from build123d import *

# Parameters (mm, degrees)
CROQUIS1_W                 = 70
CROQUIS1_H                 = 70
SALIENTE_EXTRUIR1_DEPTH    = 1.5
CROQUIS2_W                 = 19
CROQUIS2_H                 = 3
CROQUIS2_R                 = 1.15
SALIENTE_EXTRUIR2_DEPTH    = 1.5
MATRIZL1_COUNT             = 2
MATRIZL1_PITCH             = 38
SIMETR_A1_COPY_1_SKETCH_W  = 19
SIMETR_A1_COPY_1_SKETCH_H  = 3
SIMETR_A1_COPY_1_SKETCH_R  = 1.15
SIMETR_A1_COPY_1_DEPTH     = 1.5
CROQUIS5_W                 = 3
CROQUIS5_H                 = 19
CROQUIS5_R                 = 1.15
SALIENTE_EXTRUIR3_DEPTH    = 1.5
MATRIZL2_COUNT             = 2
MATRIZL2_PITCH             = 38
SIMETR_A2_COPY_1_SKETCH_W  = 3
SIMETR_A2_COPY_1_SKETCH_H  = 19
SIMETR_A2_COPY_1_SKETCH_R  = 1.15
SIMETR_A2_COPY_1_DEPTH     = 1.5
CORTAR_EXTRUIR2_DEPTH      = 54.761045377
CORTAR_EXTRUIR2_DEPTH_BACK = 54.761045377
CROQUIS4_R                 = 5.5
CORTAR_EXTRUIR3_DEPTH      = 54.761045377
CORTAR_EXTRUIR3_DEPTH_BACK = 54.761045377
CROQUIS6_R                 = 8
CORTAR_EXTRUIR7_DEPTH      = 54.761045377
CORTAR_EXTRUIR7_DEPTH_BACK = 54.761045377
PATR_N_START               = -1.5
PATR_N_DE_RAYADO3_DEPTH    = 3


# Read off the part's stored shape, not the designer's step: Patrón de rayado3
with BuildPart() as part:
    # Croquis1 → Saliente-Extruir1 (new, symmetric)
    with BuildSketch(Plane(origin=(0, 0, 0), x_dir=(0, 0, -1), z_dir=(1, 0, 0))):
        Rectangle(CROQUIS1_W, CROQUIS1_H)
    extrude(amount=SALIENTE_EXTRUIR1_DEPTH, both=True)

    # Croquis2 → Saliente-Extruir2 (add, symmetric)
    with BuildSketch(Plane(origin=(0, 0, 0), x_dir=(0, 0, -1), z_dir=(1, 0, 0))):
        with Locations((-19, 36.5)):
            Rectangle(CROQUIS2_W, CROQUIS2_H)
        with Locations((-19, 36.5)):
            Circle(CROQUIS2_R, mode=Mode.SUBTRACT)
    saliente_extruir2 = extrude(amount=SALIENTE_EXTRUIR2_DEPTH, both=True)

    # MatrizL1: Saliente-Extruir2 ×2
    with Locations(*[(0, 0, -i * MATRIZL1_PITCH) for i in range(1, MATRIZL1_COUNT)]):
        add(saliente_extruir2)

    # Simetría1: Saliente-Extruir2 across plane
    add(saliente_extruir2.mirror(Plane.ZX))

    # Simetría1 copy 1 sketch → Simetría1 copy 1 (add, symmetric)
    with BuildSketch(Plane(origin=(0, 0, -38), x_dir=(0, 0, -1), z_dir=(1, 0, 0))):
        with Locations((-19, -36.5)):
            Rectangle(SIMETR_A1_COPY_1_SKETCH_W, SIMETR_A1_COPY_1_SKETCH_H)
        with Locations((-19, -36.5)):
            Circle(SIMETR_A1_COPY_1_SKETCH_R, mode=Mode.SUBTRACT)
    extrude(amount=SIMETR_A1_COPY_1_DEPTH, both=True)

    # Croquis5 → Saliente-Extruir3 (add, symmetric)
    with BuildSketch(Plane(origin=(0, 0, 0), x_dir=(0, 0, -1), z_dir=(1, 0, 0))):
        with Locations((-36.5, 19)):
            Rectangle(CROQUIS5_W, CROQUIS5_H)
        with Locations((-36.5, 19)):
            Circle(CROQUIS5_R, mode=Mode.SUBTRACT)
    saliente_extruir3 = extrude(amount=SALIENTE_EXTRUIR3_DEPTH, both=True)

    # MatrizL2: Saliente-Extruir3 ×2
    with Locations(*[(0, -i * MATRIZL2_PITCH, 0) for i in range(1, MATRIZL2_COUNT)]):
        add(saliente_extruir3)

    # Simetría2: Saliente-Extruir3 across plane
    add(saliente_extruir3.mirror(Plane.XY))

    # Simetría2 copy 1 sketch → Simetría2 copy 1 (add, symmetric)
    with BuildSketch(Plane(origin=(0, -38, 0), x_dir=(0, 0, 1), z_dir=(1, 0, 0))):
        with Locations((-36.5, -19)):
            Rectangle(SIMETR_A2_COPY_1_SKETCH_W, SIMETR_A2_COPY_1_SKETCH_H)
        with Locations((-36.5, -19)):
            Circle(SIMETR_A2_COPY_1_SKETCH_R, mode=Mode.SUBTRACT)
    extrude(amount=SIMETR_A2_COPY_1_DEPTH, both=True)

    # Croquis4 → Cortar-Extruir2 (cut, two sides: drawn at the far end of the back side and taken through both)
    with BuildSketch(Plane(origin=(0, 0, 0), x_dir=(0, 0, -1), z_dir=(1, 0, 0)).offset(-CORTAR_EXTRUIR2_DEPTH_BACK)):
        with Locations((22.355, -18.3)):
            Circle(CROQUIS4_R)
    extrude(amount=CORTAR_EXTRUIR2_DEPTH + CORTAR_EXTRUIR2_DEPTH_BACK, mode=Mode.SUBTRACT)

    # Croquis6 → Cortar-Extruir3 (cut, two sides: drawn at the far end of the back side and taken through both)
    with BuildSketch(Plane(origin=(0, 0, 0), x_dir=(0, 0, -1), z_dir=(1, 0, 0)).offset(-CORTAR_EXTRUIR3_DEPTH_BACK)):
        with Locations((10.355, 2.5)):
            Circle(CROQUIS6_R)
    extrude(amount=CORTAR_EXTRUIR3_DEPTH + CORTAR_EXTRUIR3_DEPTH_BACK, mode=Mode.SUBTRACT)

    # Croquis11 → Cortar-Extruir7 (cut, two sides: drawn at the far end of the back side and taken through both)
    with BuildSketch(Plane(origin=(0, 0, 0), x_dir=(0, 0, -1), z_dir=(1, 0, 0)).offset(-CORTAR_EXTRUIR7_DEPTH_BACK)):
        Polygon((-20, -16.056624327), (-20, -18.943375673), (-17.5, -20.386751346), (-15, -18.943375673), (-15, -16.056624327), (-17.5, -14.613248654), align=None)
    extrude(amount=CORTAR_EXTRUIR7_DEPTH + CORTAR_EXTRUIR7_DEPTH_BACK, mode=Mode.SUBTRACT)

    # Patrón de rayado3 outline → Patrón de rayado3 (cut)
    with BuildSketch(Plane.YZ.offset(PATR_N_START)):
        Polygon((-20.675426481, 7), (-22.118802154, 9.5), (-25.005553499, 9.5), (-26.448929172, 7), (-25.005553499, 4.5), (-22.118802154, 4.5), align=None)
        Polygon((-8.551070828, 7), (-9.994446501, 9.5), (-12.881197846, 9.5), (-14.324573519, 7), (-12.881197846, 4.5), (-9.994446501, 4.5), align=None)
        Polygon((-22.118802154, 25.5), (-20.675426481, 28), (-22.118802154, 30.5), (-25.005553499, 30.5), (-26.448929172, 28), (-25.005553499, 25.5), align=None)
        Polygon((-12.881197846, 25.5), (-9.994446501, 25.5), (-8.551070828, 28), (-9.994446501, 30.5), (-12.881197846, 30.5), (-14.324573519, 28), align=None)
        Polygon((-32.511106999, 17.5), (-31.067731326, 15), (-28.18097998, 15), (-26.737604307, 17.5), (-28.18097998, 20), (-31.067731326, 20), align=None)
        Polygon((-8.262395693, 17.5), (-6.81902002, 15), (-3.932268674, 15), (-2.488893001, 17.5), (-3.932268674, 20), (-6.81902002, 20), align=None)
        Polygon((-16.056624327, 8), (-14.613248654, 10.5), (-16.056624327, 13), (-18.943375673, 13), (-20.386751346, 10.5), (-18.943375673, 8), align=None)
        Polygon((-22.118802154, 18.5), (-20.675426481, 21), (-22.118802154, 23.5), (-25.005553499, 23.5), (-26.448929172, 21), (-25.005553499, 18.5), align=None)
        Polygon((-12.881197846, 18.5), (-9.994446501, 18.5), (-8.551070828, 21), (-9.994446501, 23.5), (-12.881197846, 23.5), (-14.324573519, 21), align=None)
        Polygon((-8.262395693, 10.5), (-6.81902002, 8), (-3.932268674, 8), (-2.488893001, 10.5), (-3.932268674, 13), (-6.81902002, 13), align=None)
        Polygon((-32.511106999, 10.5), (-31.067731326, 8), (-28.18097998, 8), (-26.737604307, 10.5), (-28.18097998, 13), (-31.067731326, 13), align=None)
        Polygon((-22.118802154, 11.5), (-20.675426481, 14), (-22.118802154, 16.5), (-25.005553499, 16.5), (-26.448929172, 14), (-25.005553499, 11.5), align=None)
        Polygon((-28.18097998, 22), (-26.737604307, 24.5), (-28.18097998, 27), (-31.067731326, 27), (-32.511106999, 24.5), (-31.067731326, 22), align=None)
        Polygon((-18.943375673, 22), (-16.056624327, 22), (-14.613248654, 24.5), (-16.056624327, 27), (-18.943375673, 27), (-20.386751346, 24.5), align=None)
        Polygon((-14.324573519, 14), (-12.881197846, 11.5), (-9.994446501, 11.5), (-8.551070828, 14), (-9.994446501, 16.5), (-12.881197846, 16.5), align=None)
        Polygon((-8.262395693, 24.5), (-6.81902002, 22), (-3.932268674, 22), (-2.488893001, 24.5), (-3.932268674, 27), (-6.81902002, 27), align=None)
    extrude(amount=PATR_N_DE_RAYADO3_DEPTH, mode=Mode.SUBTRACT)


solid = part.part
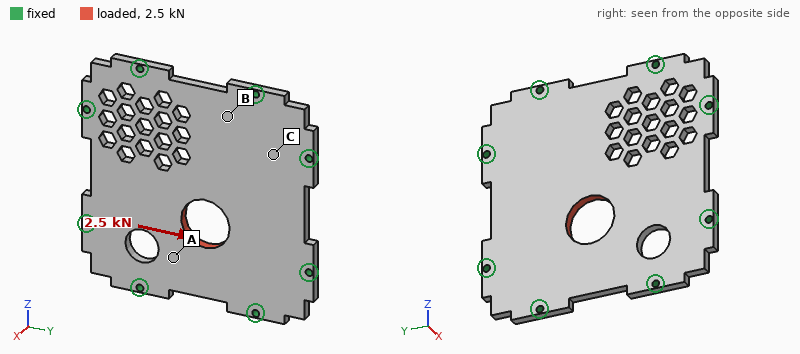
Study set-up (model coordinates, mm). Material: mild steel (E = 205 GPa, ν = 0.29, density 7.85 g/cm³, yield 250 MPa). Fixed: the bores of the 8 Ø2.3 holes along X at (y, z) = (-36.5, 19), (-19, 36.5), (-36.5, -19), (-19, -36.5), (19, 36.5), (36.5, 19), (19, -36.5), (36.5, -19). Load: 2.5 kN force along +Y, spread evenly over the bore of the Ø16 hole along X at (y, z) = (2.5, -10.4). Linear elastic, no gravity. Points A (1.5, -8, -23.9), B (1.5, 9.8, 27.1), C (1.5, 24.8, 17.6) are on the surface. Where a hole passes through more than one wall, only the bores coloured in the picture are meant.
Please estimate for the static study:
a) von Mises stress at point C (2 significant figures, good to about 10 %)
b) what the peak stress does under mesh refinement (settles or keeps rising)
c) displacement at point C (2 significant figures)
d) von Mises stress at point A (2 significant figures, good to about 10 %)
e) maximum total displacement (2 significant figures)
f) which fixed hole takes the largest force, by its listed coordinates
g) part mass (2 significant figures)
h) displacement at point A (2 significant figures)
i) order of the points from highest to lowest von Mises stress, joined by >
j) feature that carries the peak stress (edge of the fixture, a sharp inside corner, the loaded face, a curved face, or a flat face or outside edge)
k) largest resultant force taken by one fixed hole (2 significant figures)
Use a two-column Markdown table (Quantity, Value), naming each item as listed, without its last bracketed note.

| Quantity | Value |
|---|---|
| von Mises stress at point C | 8.2 MPa |
| what the peak stress does under mesh refinement | keeps rising |
| displacement at point C | 0.70 µm |
| von Mises stress at point A | 15 MPa |
| maximum total displacement | 3.0 µm |
| which fixed hole takes the largest force, by its listed coordinates | (36.5, -19) |
| part mass | 110 g |
| displacement at point A | 1.5 µm |
| order of the points from highest to lowest von Mises stress, joined by > | A > C > B |
| feature that carries the peak stress | edge of the fixture |
| largest resultant force taken by one fixed hole | 640 N |
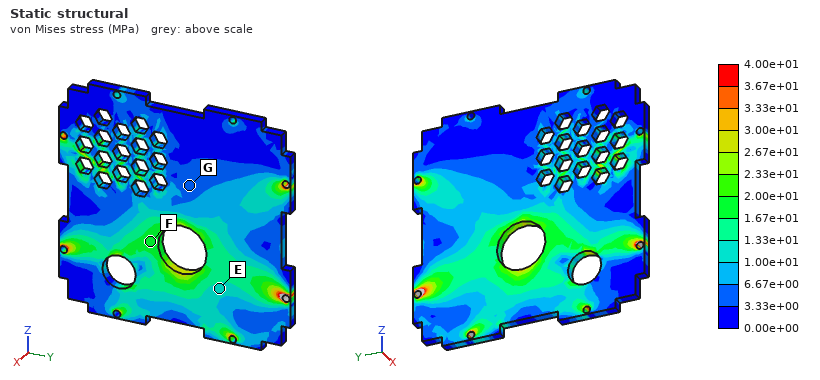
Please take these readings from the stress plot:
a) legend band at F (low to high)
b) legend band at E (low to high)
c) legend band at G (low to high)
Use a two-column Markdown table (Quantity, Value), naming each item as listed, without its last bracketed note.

| Quantity | Value |
|---|---|
| legend band at F | 1.67e+01 to 2.00e+01 MPa |
| legend band at E | 1.00e+01 to 1.33e+01 MPa |
| legend band at G | 3.33e+00 to 6.67e+00 MPa |
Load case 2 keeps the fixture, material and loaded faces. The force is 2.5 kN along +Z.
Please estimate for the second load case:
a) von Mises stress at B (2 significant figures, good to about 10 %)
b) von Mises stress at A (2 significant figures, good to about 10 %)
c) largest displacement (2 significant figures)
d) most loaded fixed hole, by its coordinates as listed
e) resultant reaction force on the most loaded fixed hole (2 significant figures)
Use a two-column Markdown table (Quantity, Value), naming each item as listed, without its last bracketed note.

| Quantity | Value |
|---|---|
| von Mises stress at B | 9.3 MPa |
| von Mises stress at A | 19 MPa |
| largest displacement | 3.4 µm |
| most loaded fixed hole, by its coordinates as listed | (19, -36.5) |
| resultant reaction force on the most loaded fixed hole | 730 N |
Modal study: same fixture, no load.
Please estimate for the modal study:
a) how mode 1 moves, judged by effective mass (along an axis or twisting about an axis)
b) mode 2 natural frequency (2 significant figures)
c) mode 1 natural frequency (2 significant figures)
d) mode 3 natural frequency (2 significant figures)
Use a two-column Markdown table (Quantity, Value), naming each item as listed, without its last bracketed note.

| Quantity | Value |
|---|---|
| how mode 1 moves, judged by effective mass | along X |
| mode 2 natural frequency | 6800 Hz |
| mode 1 natural frequency | 3300 Hz |
| mode 3 natural frequency | 7000 Hz |
